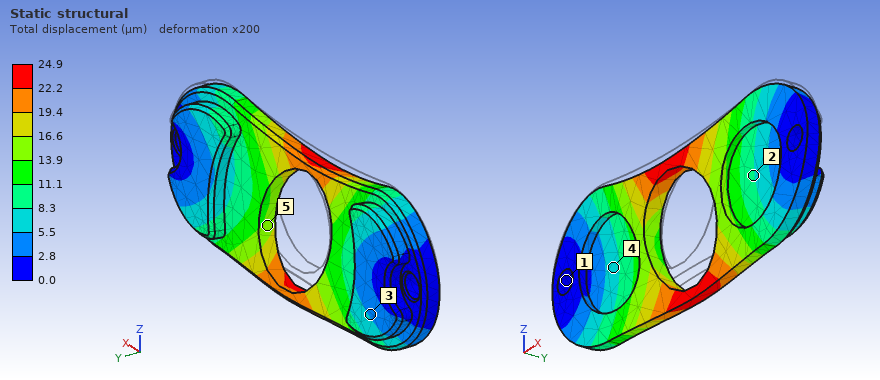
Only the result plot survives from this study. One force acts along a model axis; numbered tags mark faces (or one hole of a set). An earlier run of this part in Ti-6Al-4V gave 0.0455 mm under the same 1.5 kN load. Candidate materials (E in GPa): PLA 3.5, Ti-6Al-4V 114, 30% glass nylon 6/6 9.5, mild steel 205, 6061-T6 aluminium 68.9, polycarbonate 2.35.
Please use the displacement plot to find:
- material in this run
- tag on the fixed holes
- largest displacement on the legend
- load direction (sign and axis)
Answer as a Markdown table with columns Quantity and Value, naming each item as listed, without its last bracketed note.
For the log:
| Quantity | Value |
|---|---|
| material in this run | mild steel |
| tag on the fixed holes | 1 |
| largest displacement on the legend | 24.9 µm |
| load direction | -Z |
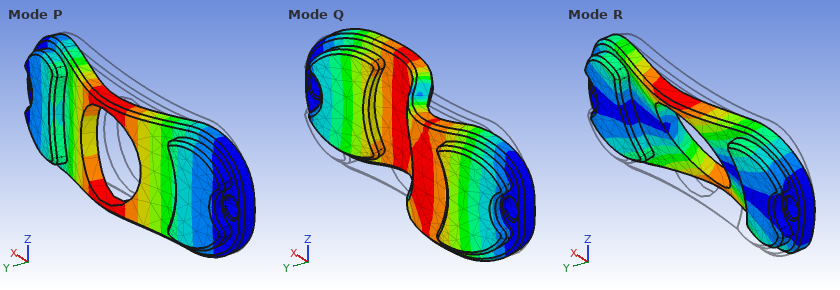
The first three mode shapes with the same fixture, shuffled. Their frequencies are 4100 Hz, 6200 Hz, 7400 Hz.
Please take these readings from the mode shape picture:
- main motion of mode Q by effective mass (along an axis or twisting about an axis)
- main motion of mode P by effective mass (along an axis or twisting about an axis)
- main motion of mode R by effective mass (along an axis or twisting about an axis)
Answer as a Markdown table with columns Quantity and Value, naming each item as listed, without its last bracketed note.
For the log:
| Quantity | Value |
|---|---|
| main motion of mode Q by effective mass | twisting about Z |
| main motion of mode P by effective mass | along Y |
| main motion of mode R by effective mass | twisting about X |
